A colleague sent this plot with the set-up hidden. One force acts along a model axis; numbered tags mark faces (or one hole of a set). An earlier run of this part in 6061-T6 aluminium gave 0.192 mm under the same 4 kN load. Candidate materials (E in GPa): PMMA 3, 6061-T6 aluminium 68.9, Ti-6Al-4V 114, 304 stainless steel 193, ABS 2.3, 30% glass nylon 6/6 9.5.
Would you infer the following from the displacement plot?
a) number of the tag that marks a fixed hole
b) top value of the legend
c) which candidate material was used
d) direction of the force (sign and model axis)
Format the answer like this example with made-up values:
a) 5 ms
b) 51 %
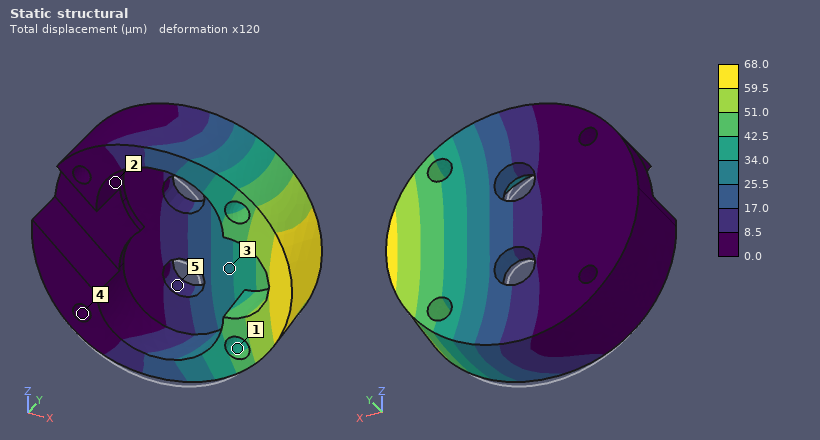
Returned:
a) 4
b) 68.0 µm
c) 304 stainless steel
d) +Y
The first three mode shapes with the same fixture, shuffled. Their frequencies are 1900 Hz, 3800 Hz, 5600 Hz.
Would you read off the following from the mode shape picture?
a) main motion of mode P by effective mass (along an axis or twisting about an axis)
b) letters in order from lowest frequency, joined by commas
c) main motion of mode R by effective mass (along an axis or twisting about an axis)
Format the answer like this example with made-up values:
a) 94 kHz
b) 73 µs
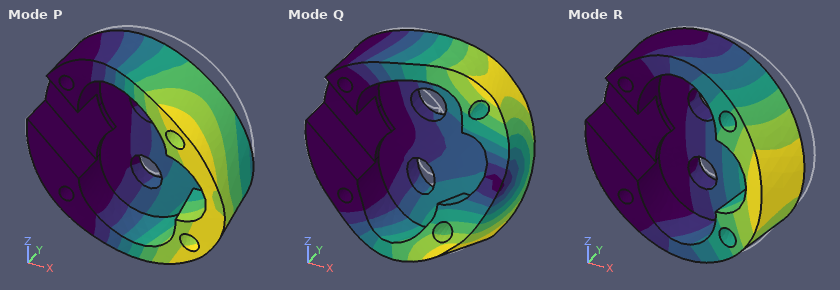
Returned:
a) along Z
b) R, P, Q
c) along Y
